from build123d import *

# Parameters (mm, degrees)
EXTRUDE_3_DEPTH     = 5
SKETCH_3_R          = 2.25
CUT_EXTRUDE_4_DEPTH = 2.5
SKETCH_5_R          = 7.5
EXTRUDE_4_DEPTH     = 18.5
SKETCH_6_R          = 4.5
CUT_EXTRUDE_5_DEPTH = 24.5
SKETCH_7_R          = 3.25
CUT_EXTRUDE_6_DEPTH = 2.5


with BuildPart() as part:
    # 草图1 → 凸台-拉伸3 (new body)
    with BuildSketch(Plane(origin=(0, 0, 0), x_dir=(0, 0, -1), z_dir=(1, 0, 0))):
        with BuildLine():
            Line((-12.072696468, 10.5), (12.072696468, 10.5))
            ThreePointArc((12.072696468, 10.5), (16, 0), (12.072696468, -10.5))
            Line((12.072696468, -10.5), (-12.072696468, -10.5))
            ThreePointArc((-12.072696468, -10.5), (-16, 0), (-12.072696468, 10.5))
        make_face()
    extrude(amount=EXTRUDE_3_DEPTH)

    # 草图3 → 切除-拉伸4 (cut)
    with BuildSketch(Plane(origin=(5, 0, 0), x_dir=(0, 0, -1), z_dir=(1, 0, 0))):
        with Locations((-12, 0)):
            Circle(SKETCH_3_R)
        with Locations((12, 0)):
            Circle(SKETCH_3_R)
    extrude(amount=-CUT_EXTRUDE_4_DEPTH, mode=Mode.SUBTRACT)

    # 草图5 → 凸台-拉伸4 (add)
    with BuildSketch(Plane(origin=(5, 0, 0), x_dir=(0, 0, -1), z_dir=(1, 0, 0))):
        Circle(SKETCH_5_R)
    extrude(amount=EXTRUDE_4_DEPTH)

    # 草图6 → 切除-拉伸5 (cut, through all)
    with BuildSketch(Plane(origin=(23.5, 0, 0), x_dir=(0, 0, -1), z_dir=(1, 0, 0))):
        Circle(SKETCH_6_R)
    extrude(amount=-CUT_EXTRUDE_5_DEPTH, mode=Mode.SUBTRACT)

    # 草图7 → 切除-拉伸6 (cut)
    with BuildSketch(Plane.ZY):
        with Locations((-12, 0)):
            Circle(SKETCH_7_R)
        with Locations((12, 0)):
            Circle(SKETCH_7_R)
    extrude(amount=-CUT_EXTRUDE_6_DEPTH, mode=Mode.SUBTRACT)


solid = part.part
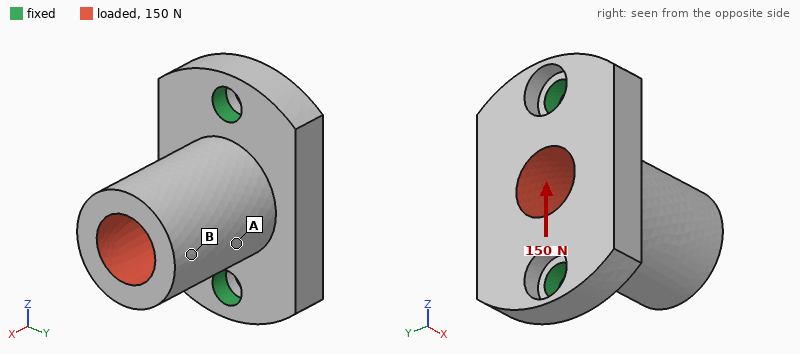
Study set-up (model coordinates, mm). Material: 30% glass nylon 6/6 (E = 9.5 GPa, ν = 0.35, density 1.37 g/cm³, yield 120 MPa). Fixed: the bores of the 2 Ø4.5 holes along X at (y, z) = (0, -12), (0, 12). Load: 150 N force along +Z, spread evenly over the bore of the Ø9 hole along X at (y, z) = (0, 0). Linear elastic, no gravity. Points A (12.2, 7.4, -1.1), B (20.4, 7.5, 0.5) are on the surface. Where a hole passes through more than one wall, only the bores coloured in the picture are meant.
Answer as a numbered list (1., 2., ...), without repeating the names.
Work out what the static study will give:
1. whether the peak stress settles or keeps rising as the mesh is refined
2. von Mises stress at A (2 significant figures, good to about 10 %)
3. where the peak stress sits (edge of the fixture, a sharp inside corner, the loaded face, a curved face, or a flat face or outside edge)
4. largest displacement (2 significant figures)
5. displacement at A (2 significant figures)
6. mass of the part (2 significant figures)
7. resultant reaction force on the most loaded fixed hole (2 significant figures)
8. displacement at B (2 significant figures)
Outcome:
1. keeps rising
2. 1.7 MPa
3. edge of the fixture
4. 21 µm
5. 9.1 µm
6. 6.3 g
7. 97 N
8. 17 µm
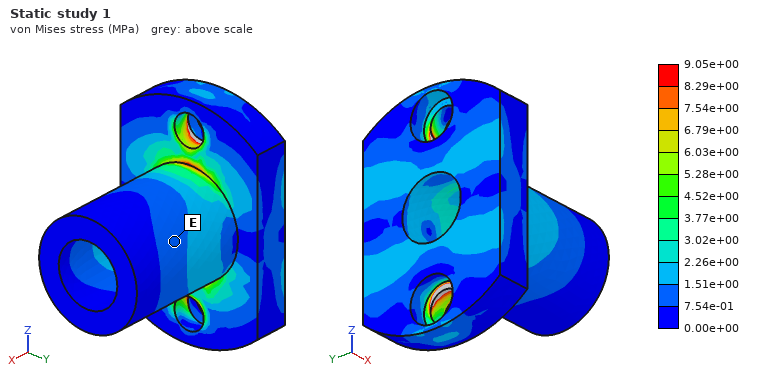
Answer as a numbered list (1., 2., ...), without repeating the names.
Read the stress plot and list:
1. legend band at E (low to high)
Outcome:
1. 7.54e-01 to 1.51e+00 MPa
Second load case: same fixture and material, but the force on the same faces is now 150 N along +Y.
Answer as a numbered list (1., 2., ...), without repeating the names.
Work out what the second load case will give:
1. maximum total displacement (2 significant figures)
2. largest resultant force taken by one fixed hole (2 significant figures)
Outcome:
1. 86 µm
2. 75 N
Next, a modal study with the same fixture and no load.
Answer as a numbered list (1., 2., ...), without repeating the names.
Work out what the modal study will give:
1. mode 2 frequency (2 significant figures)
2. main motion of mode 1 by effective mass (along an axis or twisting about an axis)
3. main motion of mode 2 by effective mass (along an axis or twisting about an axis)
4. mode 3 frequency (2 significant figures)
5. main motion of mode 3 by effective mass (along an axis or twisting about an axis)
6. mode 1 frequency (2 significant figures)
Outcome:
1. 8300 Hz
2. along Y
3. along Z
4. 10 kHz
5. along X
6. 3800 Hz
